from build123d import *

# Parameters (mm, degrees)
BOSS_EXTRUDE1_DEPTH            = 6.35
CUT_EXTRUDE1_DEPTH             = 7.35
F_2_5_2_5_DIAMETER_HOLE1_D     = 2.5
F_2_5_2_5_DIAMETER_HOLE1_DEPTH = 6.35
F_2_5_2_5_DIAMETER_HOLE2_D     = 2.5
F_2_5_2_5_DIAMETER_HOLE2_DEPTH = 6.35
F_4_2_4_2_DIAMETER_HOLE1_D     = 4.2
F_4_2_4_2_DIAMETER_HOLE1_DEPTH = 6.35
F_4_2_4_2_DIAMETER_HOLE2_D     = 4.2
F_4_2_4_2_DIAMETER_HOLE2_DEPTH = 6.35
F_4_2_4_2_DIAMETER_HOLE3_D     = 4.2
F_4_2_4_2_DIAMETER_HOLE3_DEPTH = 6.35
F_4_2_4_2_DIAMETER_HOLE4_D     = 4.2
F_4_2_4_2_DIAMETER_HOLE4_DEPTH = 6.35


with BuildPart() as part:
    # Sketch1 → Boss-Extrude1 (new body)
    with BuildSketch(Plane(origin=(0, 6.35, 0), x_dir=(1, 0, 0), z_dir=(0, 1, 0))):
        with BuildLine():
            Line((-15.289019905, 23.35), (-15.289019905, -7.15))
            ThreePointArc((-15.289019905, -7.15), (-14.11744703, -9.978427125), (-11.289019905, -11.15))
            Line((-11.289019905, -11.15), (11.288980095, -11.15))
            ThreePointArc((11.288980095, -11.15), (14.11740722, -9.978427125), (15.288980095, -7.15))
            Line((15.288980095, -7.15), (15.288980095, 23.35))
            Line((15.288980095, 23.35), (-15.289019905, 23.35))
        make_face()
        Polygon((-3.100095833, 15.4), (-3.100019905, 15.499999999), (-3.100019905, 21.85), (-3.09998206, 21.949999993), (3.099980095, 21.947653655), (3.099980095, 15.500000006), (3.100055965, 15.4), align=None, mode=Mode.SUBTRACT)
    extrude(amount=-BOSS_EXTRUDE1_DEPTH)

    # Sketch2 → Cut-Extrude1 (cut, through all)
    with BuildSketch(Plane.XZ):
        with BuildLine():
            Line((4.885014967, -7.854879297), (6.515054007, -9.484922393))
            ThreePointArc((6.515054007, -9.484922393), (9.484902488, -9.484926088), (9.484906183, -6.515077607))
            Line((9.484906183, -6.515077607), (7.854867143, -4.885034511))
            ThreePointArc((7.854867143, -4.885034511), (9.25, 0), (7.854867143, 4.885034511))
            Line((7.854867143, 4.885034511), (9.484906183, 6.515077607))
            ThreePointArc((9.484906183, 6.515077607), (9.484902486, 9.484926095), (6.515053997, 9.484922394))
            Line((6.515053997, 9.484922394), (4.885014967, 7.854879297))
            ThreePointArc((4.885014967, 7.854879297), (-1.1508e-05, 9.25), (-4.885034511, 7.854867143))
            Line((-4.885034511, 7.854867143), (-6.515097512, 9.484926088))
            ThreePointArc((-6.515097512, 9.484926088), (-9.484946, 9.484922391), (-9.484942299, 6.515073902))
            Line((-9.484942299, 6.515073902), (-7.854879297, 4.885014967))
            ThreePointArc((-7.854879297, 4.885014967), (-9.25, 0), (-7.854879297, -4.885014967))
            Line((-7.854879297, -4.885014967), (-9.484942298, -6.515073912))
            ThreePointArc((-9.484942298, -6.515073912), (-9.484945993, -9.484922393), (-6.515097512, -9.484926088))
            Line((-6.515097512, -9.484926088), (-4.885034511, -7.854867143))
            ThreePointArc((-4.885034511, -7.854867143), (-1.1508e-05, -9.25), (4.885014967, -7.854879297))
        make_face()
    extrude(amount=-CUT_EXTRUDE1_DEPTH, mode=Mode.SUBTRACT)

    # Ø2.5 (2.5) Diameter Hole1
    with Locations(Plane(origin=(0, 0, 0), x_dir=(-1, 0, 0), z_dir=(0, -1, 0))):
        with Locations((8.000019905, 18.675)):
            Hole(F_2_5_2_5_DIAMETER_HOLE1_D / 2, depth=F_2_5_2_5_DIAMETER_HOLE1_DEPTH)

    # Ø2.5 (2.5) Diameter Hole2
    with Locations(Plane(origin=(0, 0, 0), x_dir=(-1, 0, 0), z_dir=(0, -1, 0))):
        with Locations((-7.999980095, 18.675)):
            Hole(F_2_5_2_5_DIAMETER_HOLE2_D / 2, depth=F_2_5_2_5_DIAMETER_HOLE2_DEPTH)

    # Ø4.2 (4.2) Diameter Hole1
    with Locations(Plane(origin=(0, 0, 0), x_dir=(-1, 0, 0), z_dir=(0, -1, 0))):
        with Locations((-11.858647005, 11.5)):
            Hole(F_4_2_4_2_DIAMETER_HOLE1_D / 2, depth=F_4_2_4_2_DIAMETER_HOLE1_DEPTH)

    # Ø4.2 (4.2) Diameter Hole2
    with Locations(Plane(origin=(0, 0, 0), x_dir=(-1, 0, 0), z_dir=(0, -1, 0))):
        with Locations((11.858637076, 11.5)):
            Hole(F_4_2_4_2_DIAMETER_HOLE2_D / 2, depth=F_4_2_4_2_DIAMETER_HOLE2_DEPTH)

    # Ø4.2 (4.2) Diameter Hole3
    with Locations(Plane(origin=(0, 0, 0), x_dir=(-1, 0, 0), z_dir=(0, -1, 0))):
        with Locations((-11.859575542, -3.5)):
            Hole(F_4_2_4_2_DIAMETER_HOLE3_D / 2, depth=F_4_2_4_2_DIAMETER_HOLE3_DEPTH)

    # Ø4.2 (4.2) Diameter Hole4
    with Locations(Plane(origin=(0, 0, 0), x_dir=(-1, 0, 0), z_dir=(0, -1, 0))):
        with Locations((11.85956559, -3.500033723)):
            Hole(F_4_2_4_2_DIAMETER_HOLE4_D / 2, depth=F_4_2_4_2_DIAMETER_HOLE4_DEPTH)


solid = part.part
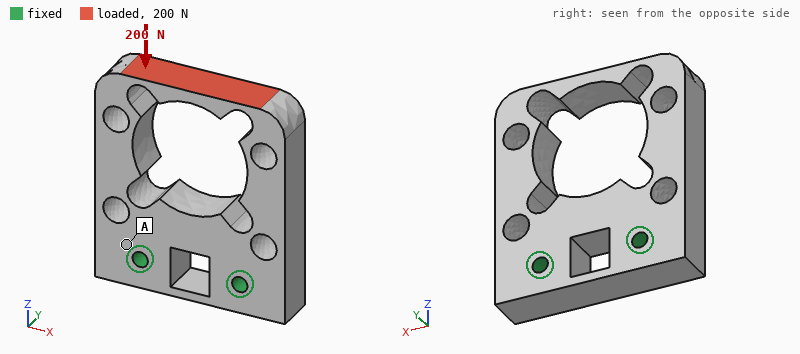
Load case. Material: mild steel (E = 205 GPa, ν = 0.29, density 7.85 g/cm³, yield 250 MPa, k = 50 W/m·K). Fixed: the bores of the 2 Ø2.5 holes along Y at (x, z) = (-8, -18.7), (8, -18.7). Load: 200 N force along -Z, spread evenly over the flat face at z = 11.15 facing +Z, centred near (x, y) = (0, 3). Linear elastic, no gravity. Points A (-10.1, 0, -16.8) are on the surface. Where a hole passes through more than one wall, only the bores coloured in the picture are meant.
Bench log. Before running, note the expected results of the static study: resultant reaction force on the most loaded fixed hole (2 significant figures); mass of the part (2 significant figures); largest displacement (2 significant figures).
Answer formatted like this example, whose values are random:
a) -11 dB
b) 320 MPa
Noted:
a) 100 N
b) 30 g
c) 11 µm
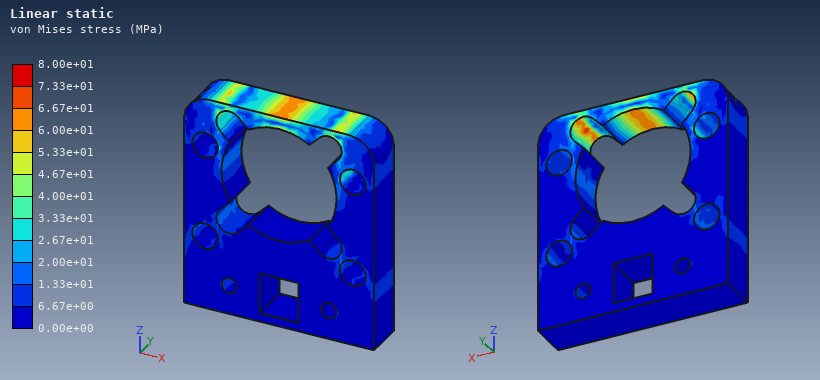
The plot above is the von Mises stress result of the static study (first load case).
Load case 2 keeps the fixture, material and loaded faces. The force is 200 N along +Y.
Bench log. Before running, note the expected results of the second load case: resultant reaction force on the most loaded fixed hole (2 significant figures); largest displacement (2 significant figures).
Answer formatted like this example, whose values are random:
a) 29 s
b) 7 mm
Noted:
a) 100 N
b) 53 µm
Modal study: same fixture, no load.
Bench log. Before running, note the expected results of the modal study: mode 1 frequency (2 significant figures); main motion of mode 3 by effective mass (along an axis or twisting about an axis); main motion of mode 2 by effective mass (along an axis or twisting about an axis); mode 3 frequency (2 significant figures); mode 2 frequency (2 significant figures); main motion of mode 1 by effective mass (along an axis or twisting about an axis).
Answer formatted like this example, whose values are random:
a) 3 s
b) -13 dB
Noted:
a) 4500 Hz
b) twisting about Z
c) along X
d) 7600 Hz
e) 5700 Hz
f) along Y
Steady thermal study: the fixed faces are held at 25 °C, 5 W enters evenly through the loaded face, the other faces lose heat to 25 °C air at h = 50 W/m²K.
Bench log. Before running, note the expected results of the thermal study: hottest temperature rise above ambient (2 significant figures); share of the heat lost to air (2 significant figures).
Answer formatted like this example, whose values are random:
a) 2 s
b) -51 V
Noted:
a) 59 K
b) 40 %
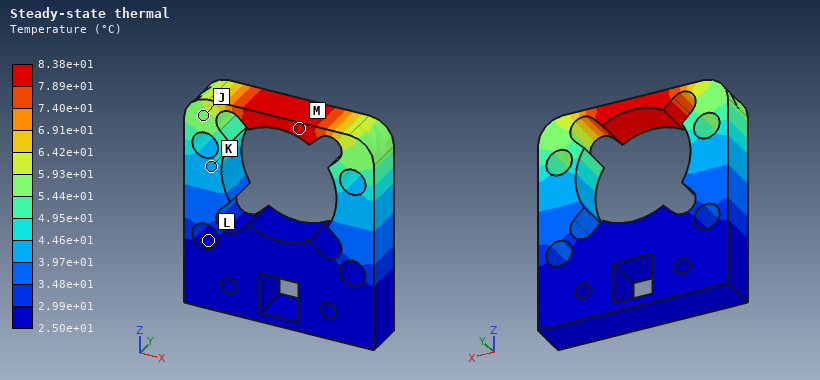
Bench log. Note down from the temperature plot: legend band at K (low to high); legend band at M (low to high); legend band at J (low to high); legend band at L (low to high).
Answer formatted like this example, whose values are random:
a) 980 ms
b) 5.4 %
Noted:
a) 3.97e+01 to 4.46e+01 °C
b) 7.89e+01 to 8.38e+01 °C
c) 5.44e+01 to 5.93e+01 °C
d) 2.50e+01 to 2.99e+01 °C
